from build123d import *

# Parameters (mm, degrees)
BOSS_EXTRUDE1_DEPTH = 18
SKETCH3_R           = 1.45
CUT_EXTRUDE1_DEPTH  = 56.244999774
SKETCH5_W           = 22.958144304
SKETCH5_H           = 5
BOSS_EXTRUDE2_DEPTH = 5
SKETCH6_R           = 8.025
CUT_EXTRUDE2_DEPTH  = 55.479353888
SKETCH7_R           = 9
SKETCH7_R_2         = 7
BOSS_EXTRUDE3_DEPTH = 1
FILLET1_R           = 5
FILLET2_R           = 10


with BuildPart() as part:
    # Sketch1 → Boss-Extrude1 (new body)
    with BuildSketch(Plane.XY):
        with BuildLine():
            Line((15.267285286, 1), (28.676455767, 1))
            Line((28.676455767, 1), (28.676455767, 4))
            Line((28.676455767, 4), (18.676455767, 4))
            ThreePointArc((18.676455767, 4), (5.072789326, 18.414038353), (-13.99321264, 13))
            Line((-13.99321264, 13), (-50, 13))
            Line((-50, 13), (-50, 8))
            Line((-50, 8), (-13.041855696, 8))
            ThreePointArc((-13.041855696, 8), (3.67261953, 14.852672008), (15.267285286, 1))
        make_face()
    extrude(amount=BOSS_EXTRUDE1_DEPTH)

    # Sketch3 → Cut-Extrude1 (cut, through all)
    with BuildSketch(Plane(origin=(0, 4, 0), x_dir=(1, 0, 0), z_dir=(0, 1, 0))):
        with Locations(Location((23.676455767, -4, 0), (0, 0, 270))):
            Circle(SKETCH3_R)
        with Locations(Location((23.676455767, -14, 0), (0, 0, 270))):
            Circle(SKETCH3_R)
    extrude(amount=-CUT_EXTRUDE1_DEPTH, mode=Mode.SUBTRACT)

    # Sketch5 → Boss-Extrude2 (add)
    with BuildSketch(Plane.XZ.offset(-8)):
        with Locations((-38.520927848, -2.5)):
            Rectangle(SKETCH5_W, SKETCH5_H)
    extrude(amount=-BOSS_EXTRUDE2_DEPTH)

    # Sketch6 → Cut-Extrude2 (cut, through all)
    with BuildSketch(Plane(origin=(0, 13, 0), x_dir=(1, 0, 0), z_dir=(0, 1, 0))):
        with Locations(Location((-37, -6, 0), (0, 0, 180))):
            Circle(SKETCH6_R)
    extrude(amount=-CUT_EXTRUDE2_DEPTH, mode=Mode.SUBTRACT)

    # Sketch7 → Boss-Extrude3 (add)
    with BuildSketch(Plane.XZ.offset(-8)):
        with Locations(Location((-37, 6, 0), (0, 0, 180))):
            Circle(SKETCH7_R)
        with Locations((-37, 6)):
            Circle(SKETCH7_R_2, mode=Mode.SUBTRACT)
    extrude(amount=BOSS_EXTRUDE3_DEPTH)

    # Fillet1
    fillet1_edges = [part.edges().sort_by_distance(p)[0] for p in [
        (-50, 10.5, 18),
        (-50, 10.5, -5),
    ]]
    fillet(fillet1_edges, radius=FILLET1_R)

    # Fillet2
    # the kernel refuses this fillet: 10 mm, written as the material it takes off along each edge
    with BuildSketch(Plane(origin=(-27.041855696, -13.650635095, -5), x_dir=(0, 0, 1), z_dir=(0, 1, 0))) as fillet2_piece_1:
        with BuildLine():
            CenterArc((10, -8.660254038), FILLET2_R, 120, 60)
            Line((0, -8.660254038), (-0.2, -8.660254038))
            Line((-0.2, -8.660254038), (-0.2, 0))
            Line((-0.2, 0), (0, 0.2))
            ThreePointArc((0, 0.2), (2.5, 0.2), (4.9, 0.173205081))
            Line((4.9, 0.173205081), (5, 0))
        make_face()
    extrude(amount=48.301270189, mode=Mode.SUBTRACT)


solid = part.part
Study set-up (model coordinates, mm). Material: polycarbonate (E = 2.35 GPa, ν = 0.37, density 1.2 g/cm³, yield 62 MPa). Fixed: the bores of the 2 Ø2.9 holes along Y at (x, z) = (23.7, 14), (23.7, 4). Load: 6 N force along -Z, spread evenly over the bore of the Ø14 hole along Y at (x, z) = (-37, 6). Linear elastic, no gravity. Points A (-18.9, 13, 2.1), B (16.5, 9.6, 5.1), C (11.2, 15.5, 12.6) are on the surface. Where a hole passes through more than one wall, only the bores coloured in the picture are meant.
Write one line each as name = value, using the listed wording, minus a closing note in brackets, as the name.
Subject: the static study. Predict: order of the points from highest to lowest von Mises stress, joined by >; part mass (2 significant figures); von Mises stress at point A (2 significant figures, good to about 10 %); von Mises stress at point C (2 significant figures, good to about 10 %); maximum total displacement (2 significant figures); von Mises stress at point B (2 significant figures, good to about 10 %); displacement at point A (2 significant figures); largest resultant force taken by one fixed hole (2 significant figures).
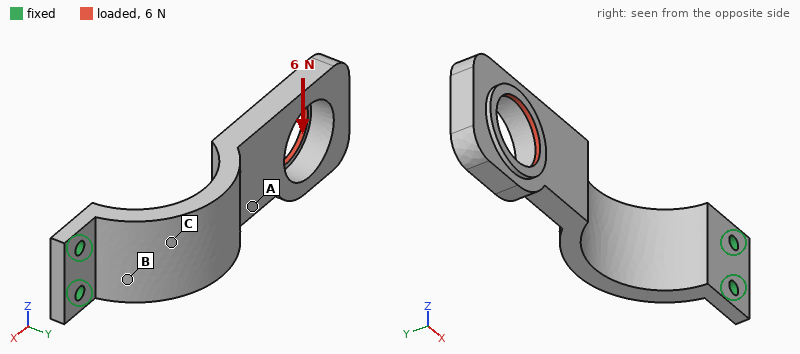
order of the points from highest to lowest von Mises stress, joined by > = B > C > A
part mass = 7.4 g
von Mises stress at point A = 0.56 MPa
von Mises stress at point C = 3.9 MPa
maximum total displacement = 0.96 mm
von Mises stress at point B = 4.7 MPa
displacement at point A = 0.44 mm
largest resultant force taken by one fixed hole = 32 N
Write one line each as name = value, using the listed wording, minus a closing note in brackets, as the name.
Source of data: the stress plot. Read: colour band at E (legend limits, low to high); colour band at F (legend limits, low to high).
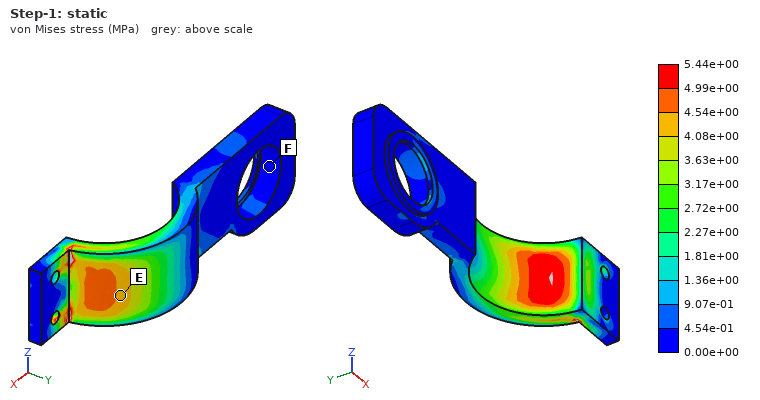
colour band at E = 4.08e+00 to 4.54e+00 MPa
colour band at F = 0.00e+00 to 4.54e-01 MPa
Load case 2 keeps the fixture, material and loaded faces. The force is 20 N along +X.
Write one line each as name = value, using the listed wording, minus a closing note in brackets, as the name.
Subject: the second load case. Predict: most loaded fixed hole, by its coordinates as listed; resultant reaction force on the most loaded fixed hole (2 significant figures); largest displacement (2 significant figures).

most loaded fixed hole, by its coordinates as listed = (23.7, 4)
resultant reaction force on the most loaded fixed hole = 15 N
largest displacement = 0.88 mm
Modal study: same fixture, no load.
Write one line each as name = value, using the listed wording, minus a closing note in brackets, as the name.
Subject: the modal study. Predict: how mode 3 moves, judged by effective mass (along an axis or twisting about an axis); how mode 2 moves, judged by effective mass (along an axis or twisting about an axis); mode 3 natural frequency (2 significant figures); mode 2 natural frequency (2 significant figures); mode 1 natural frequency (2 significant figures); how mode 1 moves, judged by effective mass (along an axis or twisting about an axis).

how mode 3 moves, judged by effective mass = along X
how mode 2 moves, judged by effective mass = along Z
mode 3 natural frequency = 630 Hz
mode 2 natural frequency = 270 Hz
mode 1 natural frequency = 120 Hz
how mode 1 moves, judged by effective mass = along Y
